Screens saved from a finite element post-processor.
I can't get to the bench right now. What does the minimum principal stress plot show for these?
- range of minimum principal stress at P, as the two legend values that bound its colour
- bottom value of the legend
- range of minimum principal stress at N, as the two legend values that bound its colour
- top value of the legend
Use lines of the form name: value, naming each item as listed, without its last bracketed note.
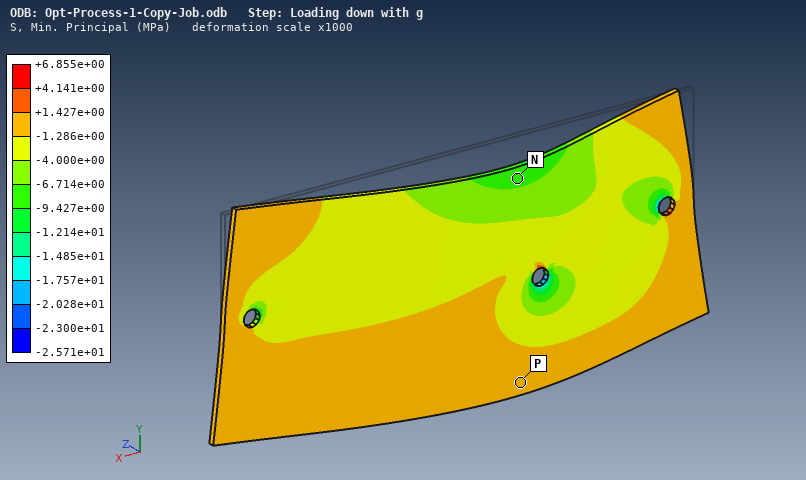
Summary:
range of minimum principal stress at P, as the two legend values that bound its colour: -1.286e+00 to +1.427e+00 MPa
bottom value of the legend: -2.571e+01 MPa
range of minimum principal stress at N, as the two legend values that bound its colour: -9.427e+00 to -6.714e+00 MPa
top value of the legend: +6.855e+00 MPa
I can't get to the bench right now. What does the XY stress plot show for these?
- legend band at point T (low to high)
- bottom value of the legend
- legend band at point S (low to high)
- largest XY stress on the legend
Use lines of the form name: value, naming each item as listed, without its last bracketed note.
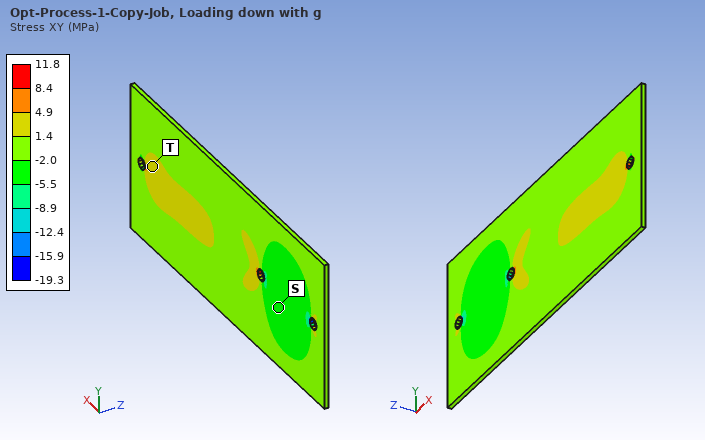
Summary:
legend band at point T: 1.4 to 4.9 MPa
bottom value of the legend: -19.3 MPa
legend band at point S: -5.5 to -2.0 MPa
largest XY stress on the legend: 11.8 MPa
